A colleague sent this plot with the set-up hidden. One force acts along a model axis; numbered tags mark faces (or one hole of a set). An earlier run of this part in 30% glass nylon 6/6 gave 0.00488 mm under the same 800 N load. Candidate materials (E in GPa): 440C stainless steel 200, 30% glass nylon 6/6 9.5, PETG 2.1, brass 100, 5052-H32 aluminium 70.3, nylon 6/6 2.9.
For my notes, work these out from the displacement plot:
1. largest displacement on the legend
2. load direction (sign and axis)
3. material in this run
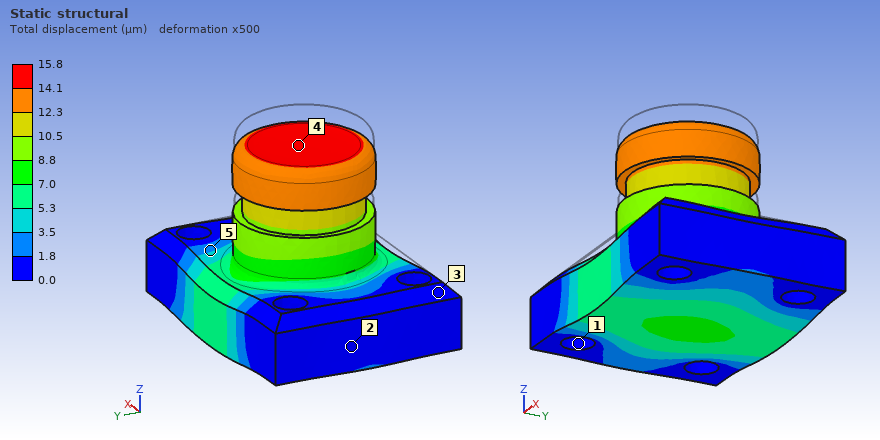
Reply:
15.8 µm
-Z
nylon 6/6
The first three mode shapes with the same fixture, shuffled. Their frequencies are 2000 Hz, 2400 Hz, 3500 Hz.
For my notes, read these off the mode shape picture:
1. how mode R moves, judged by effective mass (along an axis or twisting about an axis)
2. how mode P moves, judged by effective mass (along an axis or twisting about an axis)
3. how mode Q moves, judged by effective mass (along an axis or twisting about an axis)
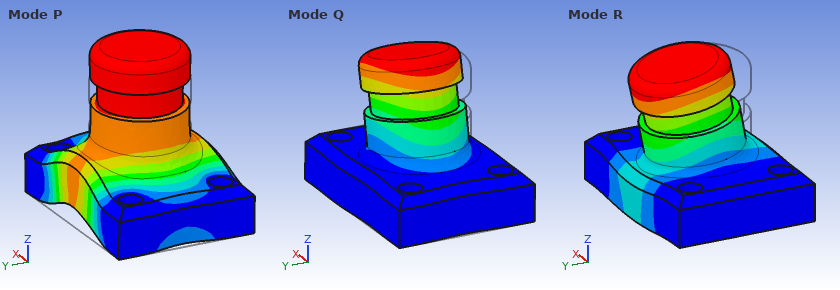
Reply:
along Y
along Z
along X
